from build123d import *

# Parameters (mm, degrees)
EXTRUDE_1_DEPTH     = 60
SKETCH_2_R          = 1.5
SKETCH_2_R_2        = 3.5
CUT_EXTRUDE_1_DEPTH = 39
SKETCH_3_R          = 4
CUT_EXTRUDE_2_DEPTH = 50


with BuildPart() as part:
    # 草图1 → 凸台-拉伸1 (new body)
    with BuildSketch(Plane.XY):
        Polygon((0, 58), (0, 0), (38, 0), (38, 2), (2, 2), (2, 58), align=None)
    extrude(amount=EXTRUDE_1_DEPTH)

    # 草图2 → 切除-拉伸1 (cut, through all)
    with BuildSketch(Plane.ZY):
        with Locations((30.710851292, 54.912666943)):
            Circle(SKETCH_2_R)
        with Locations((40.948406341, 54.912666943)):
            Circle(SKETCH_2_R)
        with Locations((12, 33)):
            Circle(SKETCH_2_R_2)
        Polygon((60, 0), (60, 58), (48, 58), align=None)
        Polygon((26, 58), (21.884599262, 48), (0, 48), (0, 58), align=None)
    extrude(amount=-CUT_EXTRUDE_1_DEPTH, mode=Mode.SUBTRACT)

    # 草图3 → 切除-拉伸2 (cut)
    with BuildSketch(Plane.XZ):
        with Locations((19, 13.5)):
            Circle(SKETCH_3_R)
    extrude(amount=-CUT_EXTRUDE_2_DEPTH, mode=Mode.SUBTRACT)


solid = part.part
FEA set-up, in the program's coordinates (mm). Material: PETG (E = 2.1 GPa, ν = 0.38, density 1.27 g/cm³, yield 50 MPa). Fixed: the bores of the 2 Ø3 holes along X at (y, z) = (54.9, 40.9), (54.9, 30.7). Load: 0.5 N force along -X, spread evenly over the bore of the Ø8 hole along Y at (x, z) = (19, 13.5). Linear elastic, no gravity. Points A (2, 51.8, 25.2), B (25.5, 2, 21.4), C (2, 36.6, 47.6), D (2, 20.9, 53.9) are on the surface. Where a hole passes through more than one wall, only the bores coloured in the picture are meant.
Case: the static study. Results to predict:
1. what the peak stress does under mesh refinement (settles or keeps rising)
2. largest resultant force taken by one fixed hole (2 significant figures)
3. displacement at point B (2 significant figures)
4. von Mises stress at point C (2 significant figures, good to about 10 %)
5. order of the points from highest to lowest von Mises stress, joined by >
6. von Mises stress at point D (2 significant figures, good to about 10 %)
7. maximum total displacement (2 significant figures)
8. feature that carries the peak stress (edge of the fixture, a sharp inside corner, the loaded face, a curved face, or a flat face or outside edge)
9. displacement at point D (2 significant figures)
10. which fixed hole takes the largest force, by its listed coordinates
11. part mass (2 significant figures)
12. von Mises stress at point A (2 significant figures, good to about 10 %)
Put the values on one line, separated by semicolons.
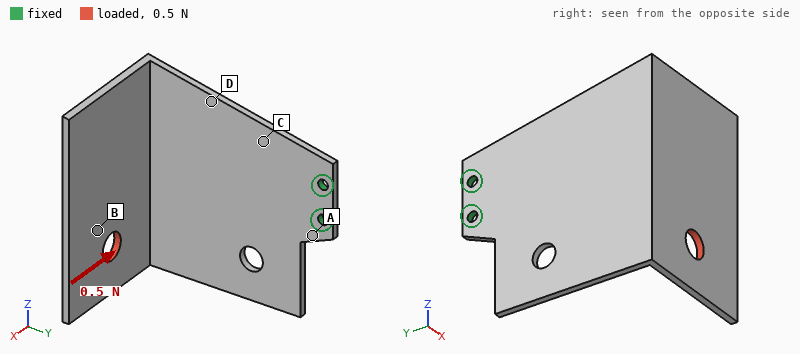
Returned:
keeps rising; 0.99 N; 0.69 mm; 0.77 MPa; A > C > D > B; 0.37 MPa; 0.92 mm; edge of the fixture; 0.17 mm; (54.9, 30.7); 13 g; 1.7 MPa
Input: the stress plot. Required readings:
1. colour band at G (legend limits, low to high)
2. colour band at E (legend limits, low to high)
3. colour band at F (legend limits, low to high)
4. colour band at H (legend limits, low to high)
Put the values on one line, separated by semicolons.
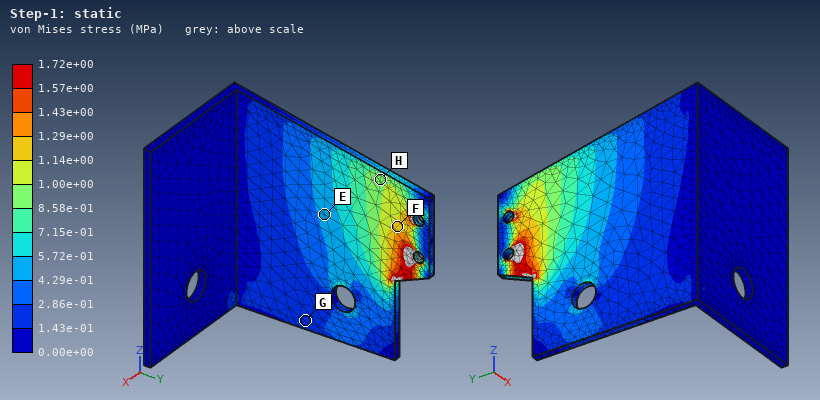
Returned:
1.43e-01 to 2.86e-01 MPa; 4.29e-01 to 5.72e-01 MPa; 1.14e+00 to 1.29e+00 MPa; 8.58e-01 to 1.00e+00 MPa
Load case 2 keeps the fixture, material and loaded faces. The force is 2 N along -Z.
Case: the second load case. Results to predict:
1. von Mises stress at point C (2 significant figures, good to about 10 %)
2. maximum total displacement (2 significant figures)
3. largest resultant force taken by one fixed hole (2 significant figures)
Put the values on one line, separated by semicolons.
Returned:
1.2 MPa; 0.98 mm; 8.7 N
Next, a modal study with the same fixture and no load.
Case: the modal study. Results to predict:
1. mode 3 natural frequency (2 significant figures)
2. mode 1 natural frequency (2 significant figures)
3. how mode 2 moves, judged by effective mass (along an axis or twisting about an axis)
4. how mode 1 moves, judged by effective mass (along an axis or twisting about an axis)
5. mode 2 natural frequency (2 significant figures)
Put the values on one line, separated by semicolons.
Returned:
200 Hz; 51 Hz; along Z; along X; 97 Hz
